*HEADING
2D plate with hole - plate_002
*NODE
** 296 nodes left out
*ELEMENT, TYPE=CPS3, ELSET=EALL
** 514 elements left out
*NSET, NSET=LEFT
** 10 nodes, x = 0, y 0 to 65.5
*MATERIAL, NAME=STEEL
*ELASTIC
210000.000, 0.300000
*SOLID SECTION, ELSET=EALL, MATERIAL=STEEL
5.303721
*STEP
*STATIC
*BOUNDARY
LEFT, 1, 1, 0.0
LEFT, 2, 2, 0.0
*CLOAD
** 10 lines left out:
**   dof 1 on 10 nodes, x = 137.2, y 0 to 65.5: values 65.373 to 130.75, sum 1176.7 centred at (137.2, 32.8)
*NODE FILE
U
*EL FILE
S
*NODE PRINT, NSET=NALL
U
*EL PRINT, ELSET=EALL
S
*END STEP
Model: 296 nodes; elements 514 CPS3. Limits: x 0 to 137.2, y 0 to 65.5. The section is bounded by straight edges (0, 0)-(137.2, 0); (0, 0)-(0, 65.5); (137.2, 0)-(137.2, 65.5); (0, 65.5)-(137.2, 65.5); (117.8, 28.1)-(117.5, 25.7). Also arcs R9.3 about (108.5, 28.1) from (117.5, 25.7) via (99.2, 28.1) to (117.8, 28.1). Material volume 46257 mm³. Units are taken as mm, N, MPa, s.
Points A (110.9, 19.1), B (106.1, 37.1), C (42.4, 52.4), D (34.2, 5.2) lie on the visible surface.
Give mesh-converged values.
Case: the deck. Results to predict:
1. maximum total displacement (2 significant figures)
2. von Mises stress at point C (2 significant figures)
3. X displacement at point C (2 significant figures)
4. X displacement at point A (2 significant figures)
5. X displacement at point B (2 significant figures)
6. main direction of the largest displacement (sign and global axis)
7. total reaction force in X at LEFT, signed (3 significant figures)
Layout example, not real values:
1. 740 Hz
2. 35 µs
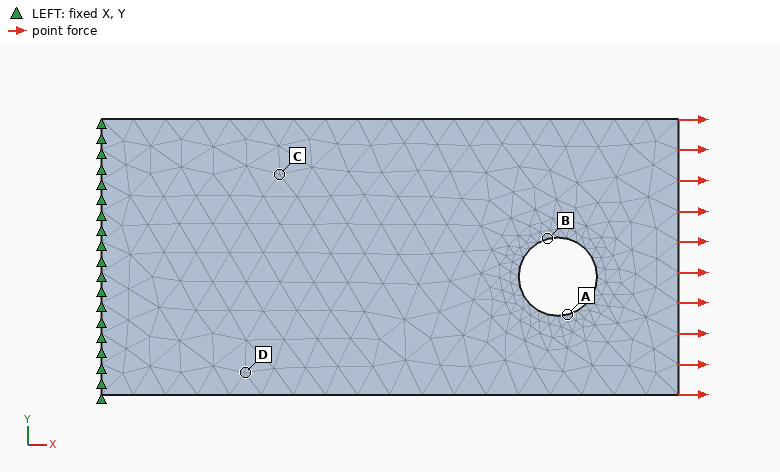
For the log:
1. 0.0028 mm
2. 3.4 MPa
3. 6.7e-04 mm
4. 0.0020 mm
5. 0.0017 mm
6. +X
7. -1180 N
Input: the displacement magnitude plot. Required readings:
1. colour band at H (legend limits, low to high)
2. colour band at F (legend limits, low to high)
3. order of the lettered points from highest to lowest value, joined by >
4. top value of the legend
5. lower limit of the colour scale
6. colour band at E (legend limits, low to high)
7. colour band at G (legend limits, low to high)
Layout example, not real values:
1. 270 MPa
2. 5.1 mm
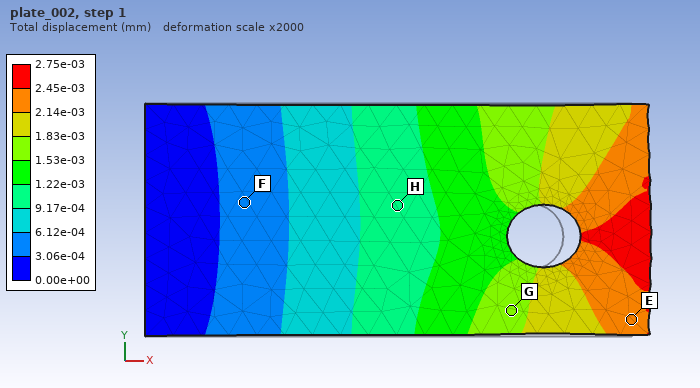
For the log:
1. 9.17e-04 to 1.22e-03 mm
2. 3.06e-04 to 6.12e-04 mm
3. E > G > H > F
4. 2.75e-03 mm
5. 0.00e+00 mm
6. 2.14e-03 to 2.45e-03 mm
7. 1.53e-03 to 1.83e-03 mm
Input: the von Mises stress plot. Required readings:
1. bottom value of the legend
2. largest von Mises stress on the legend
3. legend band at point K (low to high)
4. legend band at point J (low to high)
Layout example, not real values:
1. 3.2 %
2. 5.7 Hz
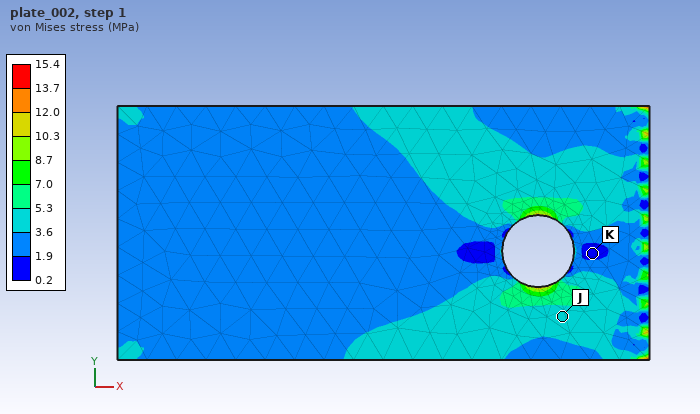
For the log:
1. 0.2 MPa
2. 15.4 MPa
3. 0.2 to 1.9 MPa
4. 3.6 to 5.3 MPa
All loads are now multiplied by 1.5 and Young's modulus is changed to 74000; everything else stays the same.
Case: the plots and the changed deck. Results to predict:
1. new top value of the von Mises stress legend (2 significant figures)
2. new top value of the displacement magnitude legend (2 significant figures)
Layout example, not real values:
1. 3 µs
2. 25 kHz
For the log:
1. 23 MPa
2. 0.012 mm
